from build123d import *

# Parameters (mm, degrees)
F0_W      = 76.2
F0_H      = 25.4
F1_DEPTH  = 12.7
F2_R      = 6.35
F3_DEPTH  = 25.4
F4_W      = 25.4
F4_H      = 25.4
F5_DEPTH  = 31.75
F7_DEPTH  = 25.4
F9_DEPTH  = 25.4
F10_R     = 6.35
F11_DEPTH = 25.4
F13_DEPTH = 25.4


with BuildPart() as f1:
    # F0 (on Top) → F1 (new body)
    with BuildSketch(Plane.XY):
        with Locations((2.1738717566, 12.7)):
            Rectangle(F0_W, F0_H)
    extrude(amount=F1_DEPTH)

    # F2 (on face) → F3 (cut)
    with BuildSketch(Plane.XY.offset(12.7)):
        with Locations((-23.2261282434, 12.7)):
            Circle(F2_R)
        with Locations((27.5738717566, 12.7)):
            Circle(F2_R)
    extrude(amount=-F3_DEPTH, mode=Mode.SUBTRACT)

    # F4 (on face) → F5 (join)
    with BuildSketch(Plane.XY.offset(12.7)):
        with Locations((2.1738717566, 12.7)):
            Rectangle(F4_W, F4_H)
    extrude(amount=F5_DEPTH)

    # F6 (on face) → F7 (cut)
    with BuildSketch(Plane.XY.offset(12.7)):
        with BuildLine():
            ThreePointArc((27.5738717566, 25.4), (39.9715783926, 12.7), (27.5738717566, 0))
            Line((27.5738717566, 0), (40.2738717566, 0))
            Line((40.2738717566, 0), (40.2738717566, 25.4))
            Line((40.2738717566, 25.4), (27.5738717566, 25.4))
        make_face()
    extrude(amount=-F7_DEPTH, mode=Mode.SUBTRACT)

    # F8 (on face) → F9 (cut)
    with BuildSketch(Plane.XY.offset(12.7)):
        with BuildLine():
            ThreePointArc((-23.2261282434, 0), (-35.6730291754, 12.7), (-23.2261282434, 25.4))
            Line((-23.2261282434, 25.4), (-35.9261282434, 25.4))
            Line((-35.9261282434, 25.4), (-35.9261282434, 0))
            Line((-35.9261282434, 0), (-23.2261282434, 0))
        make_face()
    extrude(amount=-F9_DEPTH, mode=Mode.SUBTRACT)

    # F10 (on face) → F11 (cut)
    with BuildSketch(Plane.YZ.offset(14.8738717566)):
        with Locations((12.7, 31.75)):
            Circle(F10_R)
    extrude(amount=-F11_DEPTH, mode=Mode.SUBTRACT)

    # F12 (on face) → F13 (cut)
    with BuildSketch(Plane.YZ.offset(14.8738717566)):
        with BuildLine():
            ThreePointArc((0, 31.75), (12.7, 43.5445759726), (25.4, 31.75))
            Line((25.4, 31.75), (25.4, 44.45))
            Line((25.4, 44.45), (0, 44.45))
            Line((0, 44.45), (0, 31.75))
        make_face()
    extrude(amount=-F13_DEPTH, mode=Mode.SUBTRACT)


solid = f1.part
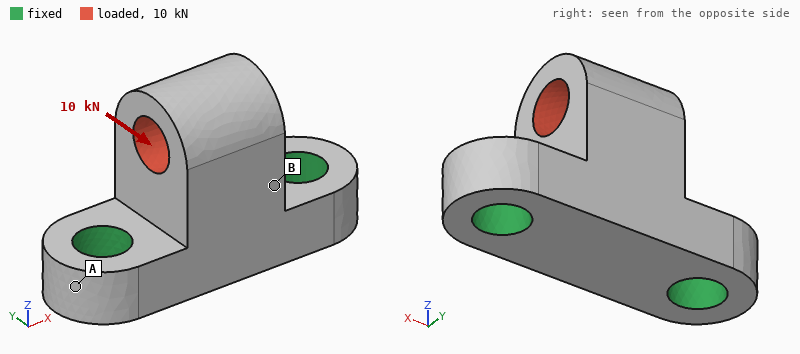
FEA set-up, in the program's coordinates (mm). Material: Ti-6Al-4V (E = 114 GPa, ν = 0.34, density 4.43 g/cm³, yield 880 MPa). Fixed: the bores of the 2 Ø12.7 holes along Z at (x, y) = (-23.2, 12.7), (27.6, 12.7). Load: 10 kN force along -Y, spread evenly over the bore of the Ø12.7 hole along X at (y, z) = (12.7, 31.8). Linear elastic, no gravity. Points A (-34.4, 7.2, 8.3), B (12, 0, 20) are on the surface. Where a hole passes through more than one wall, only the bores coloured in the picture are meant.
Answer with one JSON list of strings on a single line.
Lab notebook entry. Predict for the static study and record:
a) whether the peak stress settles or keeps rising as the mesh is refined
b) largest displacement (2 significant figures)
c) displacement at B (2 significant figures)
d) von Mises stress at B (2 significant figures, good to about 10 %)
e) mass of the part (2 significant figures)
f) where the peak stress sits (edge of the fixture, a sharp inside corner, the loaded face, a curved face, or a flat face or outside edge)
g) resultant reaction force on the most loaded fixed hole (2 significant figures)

["keeps rising", "0.13 mm", "0.058 mm", "68 MPa", "150 g", "edge of the fixture", "5.0 kN"]
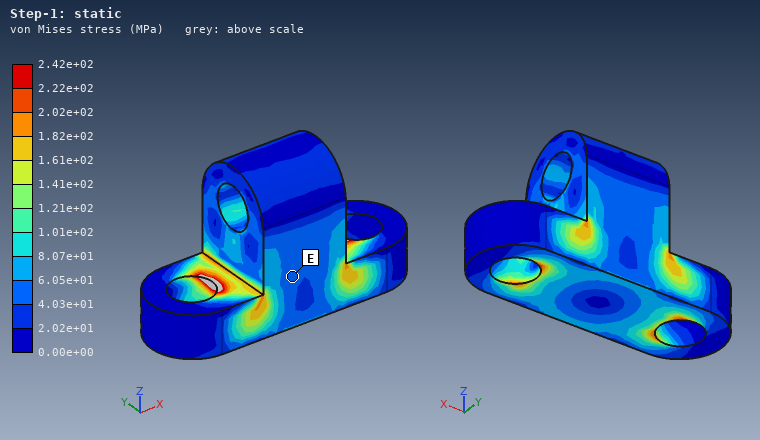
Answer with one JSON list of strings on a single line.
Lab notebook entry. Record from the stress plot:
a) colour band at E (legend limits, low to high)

["4.03e+01 to 6.05e+01 MPa"]
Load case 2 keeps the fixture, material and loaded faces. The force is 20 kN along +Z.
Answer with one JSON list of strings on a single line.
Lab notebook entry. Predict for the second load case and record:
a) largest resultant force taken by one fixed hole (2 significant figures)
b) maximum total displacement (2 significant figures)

["10 kN", "29 µm"]
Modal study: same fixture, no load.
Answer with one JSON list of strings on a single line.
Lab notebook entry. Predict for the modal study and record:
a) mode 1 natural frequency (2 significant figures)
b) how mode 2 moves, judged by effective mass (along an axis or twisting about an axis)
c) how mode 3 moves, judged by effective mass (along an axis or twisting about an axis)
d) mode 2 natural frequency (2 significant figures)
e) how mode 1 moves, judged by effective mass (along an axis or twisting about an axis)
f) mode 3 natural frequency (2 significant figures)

["7300 Hz", "along X", "along Z", "13 kHz", "along Y", "17 kHz"]
